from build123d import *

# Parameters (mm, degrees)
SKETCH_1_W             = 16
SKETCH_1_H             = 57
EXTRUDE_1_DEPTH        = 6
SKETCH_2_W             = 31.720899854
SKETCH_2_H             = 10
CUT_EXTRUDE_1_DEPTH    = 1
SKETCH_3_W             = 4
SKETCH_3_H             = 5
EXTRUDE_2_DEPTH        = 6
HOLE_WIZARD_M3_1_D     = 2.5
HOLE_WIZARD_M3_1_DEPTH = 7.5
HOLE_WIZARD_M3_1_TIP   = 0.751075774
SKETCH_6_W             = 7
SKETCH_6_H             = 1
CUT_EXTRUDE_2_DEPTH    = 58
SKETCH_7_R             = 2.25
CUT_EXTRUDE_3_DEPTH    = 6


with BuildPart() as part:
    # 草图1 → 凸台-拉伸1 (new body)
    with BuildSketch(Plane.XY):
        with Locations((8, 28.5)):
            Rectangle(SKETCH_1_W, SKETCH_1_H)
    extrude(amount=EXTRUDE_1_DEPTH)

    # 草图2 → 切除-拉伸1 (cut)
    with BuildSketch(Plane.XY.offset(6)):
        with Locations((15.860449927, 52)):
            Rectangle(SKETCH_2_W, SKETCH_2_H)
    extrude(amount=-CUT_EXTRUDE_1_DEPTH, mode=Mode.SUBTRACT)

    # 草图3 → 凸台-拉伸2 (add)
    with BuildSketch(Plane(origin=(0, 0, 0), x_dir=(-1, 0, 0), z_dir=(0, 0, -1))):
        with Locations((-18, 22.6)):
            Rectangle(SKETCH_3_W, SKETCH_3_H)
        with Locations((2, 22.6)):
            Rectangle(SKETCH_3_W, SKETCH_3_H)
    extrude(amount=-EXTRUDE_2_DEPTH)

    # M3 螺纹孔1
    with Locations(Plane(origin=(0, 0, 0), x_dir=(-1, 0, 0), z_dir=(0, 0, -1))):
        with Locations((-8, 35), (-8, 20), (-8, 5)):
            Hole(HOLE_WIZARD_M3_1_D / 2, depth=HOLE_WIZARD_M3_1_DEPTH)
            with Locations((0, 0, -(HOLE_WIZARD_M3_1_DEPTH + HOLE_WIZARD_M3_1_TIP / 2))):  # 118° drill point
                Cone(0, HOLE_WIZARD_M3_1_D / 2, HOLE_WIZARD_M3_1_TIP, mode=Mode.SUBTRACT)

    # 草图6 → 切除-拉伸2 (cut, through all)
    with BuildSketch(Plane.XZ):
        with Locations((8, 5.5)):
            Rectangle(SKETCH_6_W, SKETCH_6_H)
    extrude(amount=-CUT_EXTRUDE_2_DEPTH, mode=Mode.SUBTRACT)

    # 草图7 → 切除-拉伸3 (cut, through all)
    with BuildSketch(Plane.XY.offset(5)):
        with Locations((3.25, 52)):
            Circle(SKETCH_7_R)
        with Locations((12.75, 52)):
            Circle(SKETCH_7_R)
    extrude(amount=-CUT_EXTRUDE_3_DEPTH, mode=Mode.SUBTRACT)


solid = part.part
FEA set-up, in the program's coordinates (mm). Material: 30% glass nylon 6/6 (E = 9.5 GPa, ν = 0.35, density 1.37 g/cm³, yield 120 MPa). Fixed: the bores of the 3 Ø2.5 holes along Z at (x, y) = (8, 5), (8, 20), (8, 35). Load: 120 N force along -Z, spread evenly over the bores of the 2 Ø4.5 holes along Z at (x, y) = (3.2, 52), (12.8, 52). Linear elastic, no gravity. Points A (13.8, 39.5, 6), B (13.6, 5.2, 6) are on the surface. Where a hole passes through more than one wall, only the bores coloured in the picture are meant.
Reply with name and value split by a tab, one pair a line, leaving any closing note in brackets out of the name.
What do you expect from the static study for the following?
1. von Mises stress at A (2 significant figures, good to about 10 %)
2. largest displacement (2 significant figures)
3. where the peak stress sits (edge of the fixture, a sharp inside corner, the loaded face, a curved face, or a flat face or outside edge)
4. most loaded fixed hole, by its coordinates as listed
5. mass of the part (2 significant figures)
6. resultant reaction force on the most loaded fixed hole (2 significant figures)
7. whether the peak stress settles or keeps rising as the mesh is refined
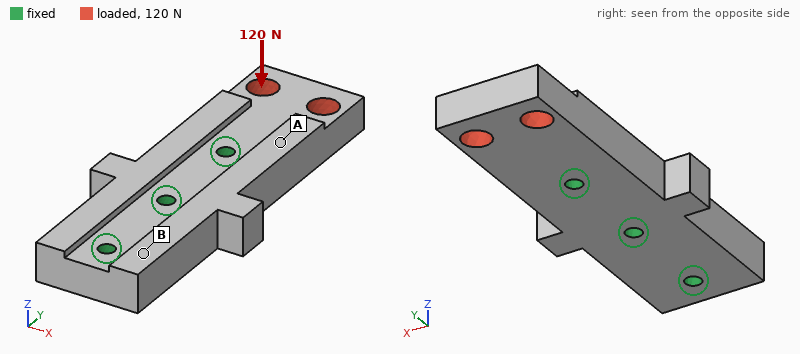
von Mises stress at A	17 MPa
largest displacement	0.17 mm
where the peak stress sits	edge of the fixture
most loaded fixed hole, by its coordinates as listed	(8, 35)
mass of the part	6.8 g
resultant reaction force on the most loaded fixed hole	180 N
whether the peak stress settles or keeps rising as the mesh is refined	keeps rising
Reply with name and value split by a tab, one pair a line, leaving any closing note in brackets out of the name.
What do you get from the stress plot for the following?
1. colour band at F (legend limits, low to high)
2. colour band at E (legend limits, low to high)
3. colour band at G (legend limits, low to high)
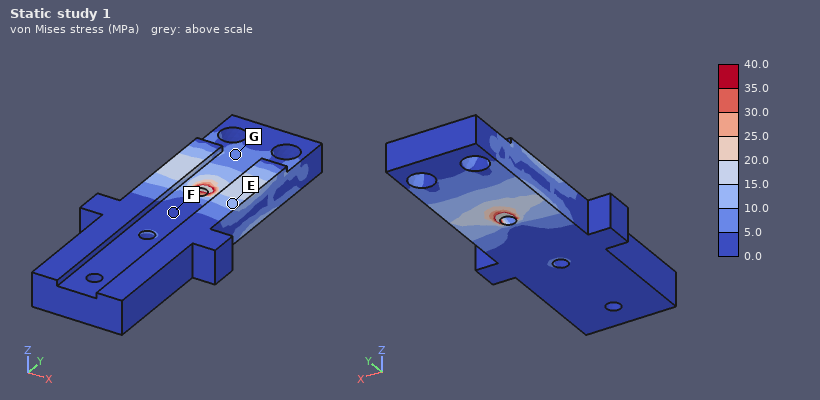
colour band at F	0.0 to 5.0 MPa
colour band at E	10.0 to 15.0 MPa
colour band at G	5.0 to 10.0 MPa
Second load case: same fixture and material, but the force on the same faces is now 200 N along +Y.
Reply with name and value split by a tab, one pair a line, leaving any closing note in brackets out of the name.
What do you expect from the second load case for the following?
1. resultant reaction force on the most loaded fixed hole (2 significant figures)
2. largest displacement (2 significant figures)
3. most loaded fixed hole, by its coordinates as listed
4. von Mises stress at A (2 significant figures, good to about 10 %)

resultant reaction force on the most loaded fixed hole	150 N
largest displacement	8.6 µm
most loaded fixed hole, by its coordinates as listed	(8, 35)
von Mises stress at A	1.2 MPa
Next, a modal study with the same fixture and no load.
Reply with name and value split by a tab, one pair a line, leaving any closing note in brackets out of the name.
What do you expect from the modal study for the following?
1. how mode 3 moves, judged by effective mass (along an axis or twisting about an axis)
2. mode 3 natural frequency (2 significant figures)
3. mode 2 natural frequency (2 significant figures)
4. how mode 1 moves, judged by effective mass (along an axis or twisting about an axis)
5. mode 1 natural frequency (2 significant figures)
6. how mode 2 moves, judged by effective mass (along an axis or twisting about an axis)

how mode 3 moves, judged by effective mass	twisting about Y
mode 3 natural frequency	9900 Hz
mode 2 natural frequency	8300 Hz
how mode 1 moves, judged by effective mass	along Z
mode 1 natural frequency	4800 Hz
how mode 2 moves, judged by effective mass	along X
